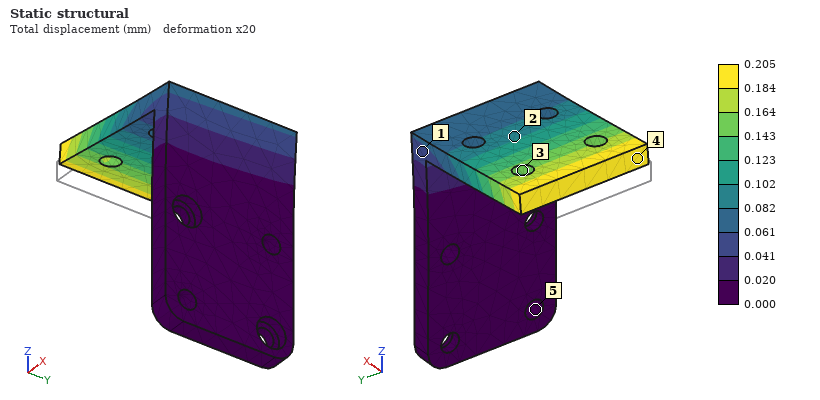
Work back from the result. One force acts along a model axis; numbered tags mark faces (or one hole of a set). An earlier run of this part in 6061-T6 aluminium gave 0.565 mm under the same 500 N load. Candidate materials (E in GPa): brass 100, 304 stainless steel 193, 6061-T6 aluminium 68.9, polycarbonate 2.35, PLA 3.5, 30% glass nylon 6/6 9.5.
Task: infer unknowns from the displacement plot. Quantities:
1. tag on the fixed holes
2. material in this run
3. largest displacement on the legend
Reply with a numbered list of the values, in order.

1. 5
2. 304 stainless steel
3. 0.205 mm
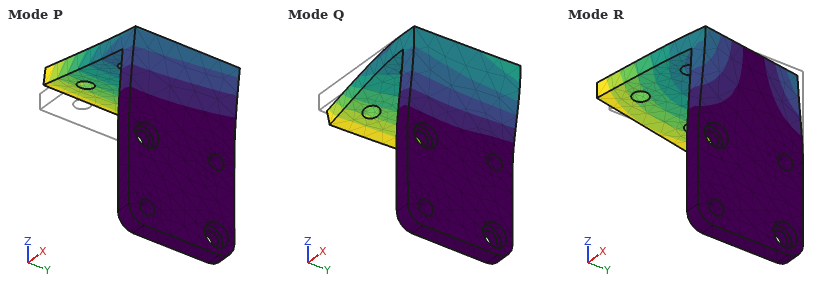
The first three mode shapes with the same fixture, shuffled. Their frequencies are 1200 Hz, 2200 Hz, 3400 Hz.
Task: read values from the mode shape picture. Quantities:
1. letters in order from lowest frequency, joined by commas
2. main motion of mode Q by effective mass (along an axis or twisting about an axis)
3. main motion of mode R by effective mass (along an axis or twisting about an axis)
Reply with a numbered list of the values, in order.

1. P, R, Q
2. along X
3. along Y
